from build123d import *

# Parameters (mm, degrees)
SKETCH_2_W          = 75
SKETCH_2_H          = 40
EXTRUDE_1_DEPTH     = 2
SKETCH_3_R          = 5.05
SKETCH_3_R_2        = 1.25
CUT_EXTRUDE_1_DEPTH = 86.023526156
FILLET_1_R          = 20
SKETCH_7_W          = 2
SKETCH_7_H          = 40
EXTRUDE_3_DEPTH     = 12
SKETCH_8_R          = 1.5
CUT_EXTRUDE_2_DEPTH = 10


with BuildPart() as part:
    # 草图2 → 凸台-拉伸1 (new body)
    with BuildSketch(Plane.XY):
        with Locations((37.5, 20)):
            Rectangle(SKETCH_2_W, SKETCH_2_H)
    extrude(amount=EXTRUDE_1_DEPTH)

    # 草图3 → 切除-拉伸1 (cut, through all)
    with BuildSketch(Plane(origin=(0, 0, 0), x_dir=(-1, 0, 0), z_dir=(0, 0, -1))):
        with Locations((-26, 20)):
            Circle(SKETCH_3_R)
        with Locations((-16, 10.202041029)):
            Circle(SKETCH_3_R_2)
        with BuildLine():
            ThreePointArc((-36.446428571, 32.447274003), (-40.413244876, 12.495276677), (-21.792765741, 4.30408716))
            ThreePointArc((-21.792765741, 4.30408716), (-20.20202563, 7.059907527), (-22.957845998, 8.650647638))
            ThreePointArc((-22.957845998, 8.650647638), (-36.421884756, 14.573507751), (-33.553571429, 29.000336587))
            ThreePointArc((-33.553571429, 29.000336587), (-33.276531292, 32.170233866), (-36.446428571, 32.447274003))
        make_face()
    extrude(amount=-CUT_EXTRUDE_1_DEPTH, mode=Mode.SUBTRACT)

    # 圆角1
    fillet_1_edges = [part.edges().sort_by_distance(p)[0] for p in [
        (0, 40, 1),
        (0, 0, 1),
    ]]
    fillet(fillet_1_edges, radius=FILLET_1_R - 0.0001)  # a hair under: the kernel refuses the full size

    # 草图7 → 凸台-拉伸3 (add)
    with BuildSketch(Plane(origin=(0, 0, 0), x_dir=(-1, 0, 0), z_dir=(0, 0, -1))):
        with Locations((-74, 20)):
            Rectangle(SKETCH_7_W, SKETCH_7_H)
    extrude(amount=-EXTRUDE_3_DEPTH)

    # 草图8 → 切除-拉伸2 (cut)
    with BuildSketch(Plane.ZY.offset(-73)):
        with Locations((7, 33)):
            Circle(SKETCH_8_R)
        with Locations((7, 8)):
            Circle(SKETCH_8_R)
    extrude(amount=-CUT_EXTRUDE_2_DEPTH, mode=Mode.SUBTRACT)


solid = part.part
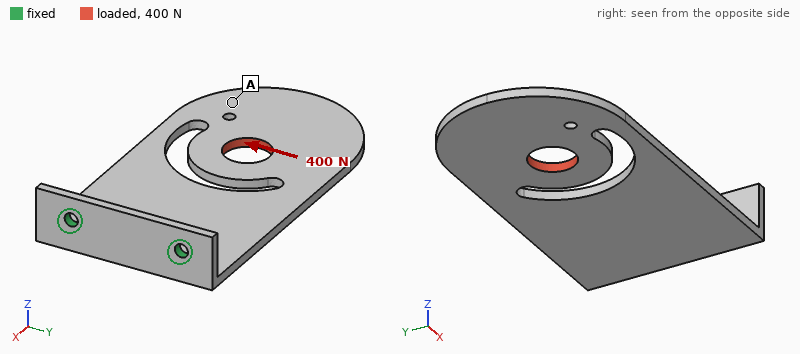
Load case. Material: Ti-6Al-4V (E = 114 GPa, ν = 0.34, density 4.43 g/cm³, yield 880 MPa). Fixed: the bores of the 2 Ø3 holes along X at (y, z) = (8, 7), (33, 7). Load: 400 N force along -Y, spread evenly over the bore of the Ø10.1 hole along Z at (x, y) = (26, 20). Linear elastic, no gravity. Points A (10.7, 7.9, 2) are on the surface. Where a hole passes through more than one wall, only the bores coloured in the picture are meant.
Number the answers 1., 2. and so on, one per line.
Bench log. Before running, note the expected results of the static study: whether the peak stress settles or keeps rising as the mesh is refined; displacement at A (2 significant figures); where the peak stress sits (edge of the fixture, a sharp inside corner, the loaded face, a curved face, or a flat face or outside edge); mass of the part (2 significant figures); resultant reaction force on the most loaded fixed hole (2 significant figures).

1. keeps rising
2. 0.22 mm
3. edge of the fixture
4. 26 g
5. 760 N
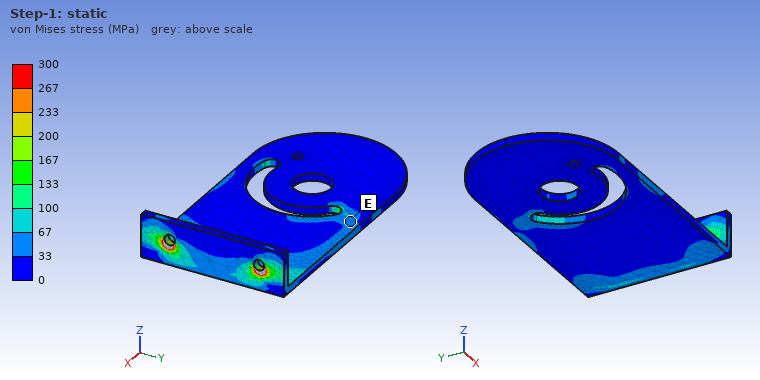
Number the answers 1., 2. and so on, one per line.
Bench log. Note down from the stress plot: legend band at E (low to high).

1. 33 to 67 MPa
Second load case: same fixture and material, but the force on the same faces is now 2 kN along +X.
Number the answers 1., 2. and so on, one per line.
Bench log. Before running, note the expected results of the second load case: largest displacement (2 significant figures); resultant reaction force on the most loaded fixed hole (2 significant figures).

1. 0.96 mm
2. 1.0 kN
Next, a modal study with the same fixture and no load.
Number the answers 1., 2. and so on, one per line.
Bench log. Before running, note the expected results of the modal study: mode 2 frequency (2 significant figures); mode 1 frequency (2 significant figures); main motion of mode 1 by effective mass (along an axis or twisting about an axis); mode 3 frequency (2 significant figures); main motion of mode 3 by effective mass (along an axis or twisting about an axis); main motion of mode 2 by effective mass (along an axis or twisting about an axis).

1. 1200 Hz
2. 290 Hz
3. along Z
4. 1400 Hz
5. along Z
6. twisting about X
